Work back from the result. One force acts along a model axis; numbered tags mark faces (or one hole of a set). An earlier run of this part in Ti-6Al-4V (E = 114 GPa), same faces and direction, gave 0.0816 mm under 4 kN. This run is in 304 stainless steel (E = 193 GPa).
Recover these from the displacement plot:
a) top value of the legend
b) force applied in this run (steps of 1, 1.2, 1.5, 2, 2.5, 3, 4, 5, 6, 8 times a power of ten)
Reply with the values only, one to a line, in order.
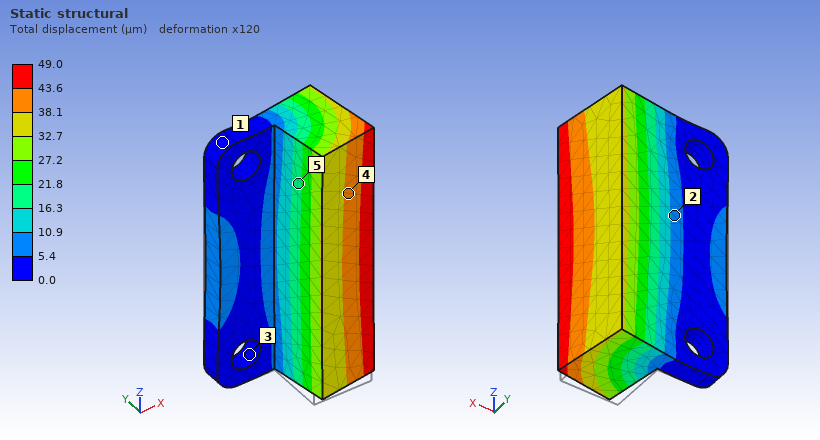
49.0 µm
4 kN
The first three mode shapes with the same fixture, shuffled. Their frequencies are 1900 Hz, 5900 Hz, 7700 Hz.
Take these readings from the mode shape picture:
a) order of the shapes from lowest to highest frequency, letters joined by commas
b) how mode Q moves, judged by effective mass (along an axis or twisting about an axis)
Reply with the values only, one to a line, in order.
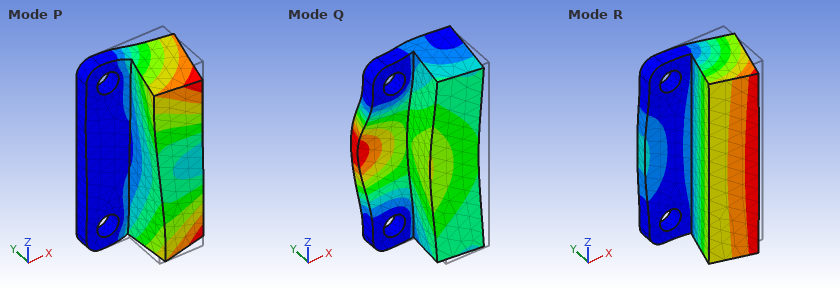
R, P, Q
along Y
